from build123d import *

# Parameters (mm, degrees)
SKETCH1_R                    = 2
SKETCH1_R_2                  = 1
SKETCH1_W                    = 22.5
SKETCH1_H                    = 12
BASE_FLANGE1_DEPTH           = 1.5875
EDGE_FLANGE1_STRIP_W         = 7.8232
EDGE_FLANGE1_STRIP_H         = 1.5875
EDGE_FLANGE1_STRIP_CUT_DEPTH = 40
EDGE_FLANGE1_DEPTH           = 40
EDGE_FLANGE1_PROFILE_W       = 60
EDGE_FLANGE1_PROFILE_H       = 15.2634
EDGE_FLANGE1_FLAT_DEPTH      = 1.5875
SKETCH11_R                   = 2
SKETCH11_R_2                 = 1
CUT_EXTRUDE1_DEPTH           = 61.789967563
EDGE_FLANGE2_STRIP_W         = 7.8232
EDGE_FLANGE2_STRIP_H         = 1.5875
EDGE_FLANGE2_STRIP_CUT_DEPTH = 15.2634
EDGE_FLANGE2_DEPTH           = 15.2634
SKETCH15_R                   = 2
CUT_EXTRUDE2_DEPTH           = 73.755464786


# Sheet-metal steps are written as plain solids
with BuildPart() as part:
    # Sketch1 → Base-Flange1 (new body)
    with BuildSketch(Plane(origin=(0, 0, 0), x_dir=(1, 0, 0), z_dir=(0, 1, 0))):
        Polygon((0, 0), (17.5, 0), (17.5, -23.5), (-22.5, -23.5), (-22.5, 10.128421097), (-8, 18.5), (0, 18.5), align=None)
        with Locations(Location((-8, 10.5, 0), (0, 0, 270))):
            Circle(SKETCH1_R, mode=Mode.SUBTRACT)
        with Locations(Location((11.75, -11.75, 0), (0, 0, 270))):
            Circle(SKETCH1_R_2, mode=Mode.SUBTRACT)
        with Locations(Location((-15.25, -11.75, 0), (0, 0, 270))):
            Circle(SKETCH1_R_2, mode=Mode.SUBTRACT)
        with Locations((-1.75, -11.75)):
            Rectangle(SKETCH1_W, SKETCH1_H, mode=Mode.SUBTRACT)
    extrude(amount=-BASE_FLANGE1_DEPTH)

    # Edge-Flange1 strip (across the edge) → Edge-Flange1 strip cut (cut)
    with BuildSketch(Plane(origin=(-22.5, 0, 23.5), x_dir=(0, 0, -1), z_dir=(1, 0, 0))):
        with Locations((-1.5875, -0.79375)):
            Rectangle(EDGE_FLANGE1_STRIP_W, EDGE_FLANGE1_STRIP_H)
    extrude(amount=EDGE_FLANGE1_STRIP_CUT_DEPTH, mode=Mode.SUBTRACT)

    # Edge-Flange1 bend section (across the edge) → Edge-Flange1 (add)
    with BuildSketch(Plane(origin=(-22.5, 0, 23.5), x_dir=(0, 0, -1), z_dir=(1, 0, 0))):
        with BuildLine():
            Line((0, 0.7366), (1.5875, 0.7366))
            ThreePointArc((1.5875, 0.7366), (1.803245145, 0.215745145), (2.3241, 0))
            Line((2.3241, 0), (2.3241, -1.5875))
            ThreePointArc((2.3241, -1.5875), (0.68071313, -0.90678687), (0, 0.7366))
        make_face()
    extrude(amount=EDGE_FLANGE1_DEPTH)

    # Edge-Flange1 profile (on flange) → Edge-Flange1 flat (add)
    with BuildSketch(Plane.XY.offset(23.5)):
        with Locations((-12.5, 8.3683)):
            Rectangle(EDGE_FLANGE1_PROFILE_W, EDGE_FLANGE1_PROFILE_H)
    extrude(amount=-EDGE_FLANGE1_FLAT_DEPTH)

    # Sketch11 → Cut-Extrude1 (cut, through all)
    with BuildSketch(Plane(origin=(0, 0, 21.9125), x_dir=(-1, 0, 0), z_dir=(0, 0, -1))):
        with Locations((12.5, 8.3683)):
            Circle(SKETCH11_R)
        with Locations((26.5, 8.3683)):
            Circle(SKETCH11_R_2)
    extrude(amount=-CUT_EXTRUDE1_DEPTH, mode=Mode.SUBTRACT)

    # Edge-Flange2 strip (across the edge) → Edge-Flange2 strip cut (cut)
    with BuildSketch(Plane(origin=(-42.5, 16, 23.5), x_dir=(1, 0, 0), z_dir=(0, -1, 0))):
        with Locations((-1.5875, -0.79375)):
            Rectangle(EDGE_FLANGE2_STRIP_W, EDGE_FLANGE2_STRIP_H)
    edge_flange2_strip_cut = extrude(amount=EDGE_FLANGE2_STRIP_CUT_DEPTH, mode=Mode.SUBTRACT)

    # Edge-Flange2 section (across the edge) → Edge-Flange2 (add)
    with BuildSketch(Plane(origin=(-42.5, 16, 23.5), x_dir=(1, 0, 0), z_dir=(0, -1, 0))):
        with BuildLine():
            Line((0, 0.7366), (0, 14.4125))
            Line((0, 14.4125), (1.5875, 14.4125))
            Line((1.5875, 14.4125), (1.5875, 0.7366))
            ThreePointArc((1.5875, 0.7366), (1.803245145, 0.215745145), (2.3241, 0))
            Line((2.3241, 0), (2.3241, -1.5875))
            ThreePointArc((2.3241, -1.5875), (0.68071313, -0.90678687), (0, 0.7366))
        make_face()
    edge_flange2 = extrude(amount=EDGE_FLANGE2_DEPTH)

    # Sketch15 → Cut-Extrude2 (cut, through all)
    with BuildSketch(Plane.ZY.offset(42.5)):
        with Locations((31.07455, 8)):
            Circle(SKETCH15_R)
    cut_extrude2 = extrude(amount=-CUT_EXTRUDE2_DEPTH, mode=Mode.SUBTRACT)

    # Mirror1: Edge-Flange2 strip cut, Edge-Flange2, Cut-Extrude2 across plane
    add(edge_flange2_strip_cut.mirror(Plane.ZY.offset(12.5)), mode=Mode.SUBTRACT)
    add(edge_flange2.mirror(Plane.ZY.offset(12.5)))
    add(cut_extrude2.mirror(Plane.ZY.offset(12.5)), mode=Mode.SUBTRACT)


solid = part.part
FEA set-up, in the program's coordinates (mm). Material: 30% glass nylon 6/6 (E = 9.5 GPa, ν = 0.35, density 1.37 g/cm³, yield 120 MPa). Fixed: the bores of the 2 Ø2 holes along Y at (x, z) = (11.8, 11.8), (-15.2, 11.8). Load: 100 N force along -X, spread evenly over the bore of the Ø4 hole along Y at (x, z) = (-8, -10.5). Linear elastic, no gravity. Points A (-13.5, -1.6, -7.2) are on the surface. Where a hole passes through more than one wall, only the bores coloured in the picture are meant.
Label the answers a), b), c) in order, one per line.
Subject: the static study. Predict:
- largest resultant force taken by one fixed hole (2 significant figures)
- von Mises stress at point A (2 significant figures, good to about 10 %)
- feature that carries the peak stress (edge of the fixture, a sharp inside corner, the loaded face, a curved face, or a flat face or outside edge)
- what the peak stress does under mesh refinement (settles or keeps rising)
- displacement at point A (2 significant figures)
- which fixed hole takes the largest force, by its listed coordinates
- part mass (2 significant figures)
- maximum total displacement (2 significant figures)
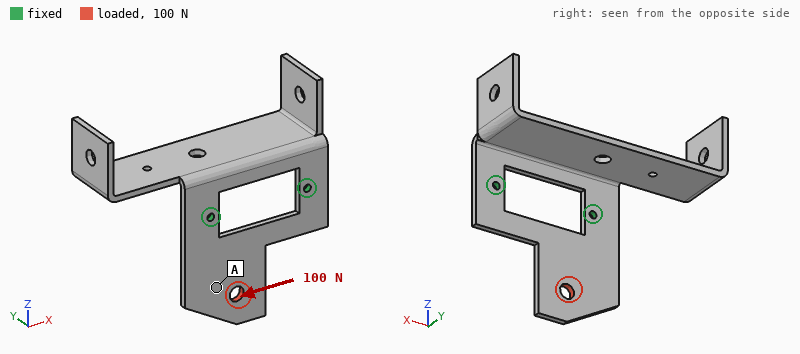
a) 94 N
b) 4.7 MPa
c) edge of the fixture
d) keeps rising
e) 0.083 mm
f) (11.8, 11.8)
g) 5.0 g
h) 0.15 mm
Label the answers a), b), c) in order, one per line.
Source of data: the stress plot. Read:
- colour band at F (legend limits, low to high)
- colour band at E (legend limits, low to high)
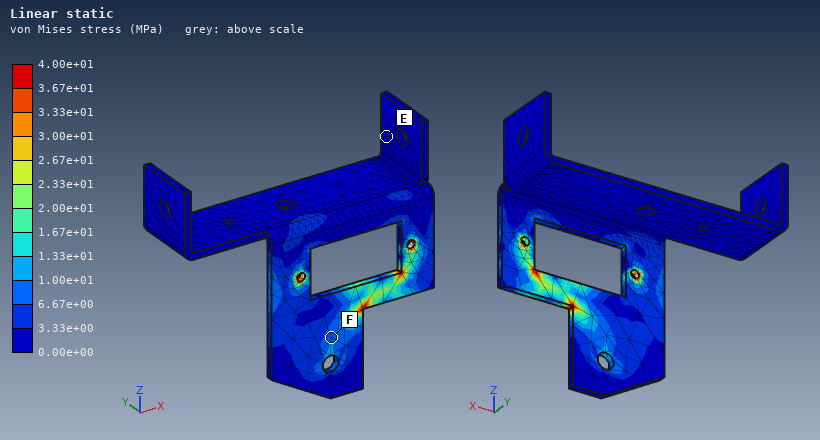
a) 6.67e+00 to 1.00e+01 MPa
b) 0.00e+00 to 3.33e+00 MPa
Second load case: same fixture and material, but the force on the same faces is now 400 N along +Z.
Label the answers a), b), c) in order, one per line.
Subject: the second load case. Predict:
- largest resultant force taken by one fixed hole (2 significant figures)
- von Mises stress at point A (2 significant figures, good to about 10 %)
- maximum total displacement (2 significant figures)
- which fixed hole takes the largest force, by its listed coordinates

a) 310 N
b) 14 MPa
c) 0.22 mm
d) (-15.2, 11.8)
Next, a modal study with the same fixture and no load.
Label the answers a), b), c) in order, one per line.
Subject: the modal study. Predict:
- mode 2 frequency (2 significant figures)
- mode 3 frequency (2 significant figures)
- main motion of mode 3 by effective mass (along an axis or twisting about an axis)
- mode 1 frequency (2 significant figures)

a) 590 Hz
b) 710 Hz
c) along Y
d) 400 Hz
